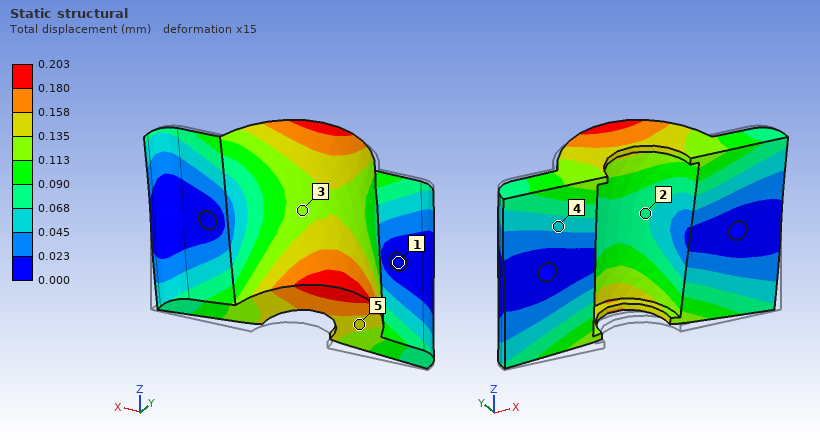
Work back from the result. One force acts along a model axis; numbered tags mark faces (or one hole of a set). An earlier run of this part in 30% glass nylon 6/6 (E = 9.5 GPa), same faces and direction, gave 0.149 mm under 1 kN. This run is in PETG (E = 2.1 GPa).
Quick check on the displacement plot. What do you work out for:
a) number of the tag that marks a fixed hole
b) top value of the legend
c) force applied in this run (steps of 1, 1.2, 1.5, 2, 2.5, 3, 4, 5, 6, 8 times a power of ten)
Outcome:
1
0.203 mm
300 N
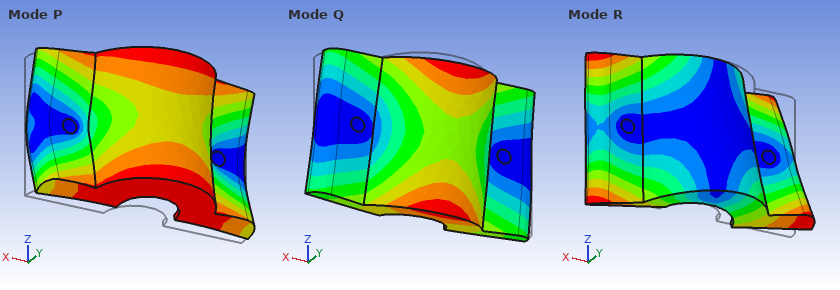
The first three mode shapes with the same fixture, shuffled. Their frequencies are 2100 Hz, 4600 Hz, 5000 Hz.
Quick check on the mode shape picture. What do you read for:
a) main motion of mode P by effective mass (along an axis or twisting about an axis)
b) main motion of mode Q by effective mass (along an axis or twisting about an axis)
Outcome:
along Y
along Z
